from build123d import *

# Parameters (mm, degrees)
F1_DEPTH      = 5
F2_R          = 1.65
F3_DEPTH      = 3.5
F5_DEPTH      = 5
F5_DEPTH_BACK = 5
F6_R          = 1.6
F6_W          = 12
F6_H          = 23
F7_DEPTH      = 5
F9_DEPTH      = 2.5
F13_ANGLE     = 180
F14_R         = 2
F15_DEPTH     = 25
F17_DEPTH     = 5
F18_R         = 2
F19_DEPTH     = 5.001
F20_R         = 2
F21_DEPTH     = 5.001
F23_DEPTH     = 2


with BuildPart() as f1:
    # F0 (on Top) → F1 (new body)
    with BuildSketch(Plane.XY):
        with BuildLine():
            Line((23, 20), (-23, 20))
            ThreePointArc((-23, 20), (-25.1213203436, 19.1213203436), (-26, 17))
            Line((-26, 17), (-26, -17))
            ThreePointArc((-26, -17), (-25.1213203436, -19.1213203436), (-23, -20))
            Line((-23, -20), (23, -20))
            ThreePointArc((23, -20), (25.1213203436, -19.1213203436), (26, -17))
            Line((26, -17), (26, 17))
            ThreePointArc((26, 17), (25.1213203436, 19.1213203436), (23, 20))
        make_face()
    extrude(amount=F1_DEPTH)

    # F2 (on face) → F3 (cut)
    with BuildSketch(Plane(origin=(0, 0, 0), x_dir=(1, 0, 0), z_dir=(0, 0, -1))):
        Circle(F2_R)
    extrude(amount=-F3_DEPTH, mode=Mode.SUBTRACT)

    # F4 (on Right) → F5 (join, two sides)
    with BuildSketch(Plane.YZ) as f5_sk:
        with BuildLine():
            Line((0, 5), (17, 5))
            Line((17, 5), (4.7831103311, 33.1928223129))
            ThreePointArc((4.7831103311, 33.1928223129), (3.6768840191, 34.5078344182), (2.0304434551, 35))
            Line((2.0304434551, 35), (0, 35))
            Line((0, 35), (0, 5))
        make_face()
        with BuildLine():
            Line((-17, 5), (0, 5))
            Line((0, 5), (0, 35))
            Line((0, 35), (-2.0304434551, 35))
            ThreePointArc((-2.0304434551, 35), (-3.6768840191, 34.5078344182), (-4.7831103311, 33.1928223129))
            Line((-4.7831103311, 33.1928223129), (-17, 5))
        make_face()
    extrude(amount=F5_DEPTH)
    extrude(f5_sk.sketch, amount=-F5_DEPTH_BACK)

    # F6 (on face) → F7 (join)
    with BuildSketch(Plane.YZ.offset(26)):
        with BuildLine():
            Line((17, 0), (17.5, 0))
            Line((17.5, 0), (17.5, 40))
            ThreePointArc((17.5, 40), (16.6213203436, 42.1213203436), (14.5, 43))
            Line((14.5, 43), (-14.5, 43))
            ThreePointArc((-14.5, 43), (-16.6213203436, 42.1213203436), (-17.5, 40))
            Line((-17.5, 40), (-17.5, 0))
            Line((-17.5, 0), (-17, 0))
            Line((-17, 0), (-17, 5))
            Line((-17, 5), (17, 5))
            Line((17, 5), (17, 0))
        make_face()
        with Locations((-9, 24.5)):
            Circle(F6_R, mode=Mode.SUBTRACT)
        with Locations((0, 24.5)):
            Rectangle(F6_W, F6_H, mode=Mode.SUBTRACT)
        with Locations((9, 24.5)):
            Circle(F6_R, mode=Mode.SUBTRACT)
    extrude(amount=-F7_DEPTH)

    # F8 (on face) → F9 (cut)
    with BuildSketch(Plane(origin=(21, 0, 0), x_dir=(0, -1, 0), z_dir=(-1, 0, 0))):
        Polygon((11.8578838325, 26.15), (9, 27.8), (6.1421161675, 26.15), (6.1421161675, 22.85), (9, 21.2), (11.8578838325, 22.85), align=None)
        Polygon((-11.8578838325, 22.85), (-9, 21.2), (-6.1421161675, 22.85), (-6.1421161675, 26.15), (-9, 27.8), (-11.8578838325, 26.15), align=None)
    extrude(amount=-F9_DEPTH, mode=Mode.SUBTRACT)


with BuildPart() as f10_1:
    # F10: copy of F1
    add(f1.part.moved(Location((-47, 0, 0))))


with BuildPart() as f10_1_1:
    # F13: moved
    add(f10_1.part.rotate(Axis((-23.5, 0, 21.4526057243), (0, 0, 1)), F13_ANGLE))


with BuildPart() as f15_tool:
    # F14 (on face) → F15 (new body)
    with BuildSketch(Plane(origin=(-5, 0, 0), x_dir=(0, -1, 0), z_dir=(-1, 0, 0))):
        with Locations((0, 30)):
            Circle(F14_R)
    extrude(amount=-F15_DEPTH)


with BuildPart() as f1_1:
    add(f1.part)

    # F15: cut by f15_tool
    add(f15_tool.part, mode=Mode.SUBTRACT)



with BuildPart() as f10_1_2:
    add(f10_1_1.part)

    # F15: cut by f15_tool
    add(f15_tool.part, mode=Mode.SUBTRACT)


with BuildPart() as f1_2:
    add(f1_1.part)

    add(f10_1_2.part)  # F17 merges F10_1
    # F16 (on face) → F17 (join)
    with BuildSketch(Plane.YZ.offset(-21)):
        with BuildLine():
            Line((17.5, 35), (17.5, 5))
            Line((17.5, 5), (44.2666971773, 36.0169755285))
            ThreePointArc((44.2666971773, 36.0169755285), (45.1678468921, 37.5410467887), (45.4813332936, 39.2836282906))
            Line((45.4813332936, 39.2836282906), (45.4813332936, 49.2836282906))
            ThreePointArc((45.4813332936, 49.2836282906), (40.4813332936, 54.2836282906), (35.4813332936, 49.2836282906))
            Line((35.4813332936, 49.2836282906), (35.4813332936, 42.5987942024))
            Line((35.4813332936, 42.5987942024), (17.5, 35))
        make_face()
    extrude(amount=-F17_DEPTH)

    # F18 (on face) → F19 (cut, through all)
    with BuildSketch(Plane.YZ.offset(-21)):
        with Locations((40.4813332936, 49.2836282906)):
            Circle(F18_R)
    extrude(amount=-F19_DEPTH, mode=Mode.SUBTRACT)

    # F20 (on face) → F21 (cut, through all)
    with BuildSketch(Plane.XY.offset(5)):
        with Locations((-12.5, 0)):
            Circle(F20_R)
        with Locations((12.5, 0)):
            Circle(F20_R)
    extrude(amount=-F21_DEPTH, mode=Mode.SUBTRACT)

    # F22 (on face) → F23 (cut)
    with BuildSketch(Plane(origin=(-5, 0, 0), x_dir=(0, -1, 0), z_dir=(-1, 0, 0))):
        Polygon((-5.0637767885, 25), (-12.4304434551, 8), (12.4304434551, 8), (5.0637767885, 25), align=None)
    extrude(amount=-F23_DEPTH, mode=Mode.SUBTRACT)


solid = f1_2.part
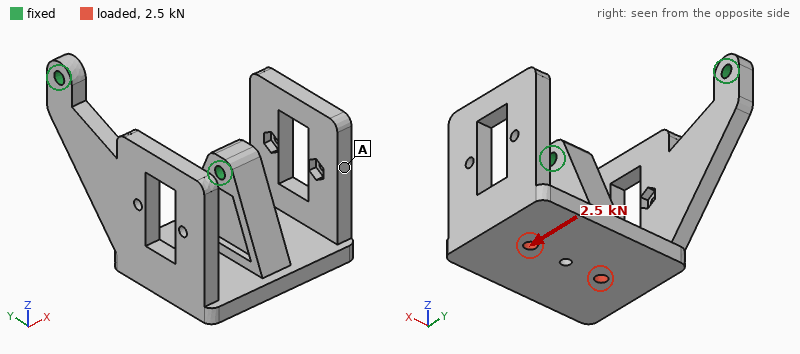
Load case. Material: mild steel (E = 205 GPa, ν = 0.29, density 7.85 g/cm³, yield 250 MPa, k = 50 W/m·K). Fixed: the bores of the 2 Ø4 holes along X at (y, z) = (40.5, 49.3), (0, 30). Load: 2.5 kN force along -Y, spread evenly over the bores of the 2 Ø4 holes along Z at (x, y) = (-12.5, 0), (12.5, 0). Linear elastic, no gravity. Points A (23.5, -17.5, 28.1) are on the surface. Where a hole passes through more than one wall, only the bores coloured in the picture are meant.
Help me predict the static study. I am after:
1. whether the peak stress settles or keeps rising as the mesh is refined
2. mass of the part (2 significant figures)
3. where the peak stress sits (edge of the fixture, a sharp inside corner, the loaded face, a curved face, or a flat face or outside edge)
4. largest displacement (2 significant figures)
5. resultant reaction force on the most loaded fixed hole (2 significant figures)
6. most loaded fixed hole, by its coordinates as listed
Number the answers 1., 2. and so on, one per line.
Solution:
1. keeps rising
2. 230 g
3. edge of the fixture
4. 93 µm
5. 2.2 kN
6. (0, 30)
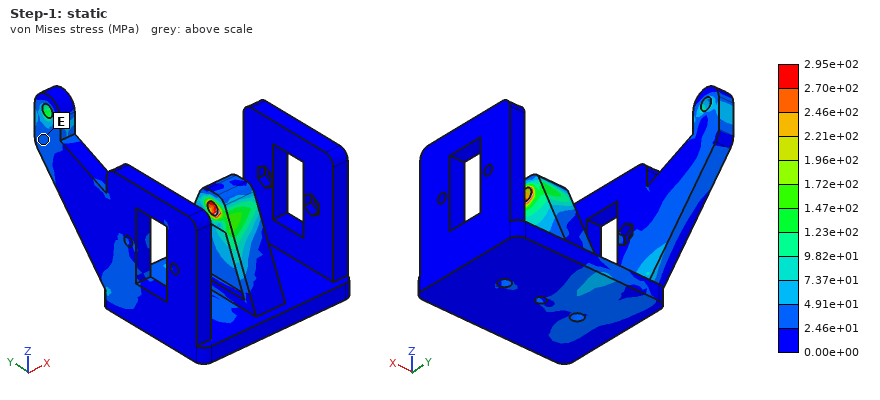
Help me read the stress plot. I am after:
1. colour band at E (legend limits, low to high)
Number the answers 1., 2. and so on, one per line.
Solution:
1. 2.46e+01 to 4.91e+01 MPa
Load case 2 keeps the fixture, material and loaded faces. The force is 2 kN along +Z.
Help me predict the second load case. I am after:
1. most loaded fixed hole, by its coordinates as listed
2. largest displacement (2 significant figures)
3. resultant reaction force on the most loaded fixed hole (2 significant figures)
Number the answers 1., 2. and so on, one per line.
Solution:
1. (0, 30)
2. 30 µm
3. 1.9 kN
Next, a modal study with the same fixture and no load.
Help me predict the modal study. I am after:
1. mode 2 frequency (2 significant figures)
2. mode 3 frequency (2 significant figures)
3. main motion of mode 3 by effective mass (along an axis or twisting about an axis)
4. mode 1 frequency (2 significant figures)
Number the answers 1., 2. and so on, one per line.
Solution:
1. 1900 Hz
2. 2300 Hz
3. along X
4. 1400 Hz
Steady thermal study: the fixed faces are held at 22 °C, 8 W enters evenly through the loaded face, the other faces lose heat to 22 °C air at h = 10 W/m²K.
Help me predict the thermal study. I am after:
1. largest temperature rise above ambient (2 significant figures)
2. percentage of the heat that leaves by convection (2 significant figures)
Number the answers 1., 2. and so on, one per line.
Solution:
1. 21 K
2. 23 %
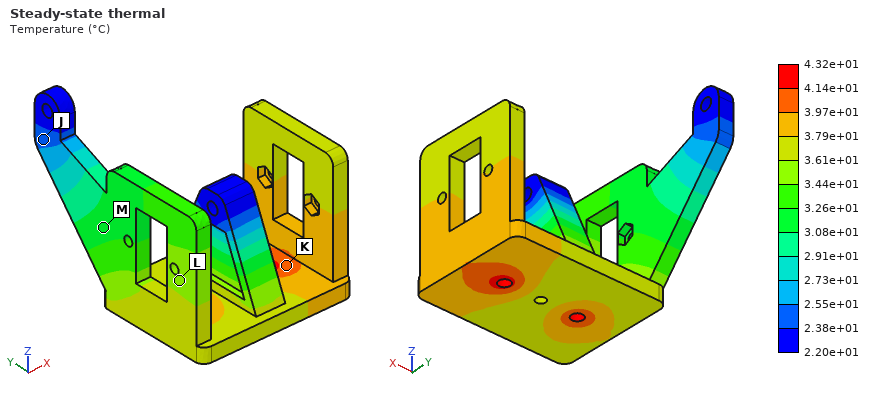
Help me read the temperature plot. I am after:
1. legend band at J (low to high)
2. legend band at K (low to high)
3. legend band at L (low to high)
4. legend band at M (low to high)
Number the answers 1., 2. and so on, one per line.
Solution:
1. 2.38e+01 to 2.55e+01 °C
2. 3.97e+01 to 4.14e+01 °C
3. 3.44e+01 to 3.61e+01 °C
4. 3.08e+01 to 3.26e+01 °C
